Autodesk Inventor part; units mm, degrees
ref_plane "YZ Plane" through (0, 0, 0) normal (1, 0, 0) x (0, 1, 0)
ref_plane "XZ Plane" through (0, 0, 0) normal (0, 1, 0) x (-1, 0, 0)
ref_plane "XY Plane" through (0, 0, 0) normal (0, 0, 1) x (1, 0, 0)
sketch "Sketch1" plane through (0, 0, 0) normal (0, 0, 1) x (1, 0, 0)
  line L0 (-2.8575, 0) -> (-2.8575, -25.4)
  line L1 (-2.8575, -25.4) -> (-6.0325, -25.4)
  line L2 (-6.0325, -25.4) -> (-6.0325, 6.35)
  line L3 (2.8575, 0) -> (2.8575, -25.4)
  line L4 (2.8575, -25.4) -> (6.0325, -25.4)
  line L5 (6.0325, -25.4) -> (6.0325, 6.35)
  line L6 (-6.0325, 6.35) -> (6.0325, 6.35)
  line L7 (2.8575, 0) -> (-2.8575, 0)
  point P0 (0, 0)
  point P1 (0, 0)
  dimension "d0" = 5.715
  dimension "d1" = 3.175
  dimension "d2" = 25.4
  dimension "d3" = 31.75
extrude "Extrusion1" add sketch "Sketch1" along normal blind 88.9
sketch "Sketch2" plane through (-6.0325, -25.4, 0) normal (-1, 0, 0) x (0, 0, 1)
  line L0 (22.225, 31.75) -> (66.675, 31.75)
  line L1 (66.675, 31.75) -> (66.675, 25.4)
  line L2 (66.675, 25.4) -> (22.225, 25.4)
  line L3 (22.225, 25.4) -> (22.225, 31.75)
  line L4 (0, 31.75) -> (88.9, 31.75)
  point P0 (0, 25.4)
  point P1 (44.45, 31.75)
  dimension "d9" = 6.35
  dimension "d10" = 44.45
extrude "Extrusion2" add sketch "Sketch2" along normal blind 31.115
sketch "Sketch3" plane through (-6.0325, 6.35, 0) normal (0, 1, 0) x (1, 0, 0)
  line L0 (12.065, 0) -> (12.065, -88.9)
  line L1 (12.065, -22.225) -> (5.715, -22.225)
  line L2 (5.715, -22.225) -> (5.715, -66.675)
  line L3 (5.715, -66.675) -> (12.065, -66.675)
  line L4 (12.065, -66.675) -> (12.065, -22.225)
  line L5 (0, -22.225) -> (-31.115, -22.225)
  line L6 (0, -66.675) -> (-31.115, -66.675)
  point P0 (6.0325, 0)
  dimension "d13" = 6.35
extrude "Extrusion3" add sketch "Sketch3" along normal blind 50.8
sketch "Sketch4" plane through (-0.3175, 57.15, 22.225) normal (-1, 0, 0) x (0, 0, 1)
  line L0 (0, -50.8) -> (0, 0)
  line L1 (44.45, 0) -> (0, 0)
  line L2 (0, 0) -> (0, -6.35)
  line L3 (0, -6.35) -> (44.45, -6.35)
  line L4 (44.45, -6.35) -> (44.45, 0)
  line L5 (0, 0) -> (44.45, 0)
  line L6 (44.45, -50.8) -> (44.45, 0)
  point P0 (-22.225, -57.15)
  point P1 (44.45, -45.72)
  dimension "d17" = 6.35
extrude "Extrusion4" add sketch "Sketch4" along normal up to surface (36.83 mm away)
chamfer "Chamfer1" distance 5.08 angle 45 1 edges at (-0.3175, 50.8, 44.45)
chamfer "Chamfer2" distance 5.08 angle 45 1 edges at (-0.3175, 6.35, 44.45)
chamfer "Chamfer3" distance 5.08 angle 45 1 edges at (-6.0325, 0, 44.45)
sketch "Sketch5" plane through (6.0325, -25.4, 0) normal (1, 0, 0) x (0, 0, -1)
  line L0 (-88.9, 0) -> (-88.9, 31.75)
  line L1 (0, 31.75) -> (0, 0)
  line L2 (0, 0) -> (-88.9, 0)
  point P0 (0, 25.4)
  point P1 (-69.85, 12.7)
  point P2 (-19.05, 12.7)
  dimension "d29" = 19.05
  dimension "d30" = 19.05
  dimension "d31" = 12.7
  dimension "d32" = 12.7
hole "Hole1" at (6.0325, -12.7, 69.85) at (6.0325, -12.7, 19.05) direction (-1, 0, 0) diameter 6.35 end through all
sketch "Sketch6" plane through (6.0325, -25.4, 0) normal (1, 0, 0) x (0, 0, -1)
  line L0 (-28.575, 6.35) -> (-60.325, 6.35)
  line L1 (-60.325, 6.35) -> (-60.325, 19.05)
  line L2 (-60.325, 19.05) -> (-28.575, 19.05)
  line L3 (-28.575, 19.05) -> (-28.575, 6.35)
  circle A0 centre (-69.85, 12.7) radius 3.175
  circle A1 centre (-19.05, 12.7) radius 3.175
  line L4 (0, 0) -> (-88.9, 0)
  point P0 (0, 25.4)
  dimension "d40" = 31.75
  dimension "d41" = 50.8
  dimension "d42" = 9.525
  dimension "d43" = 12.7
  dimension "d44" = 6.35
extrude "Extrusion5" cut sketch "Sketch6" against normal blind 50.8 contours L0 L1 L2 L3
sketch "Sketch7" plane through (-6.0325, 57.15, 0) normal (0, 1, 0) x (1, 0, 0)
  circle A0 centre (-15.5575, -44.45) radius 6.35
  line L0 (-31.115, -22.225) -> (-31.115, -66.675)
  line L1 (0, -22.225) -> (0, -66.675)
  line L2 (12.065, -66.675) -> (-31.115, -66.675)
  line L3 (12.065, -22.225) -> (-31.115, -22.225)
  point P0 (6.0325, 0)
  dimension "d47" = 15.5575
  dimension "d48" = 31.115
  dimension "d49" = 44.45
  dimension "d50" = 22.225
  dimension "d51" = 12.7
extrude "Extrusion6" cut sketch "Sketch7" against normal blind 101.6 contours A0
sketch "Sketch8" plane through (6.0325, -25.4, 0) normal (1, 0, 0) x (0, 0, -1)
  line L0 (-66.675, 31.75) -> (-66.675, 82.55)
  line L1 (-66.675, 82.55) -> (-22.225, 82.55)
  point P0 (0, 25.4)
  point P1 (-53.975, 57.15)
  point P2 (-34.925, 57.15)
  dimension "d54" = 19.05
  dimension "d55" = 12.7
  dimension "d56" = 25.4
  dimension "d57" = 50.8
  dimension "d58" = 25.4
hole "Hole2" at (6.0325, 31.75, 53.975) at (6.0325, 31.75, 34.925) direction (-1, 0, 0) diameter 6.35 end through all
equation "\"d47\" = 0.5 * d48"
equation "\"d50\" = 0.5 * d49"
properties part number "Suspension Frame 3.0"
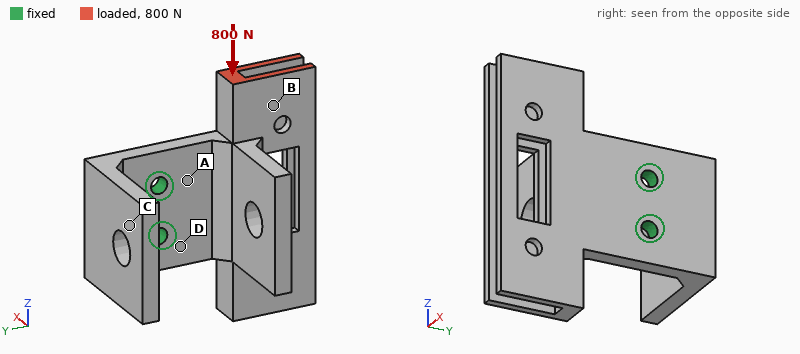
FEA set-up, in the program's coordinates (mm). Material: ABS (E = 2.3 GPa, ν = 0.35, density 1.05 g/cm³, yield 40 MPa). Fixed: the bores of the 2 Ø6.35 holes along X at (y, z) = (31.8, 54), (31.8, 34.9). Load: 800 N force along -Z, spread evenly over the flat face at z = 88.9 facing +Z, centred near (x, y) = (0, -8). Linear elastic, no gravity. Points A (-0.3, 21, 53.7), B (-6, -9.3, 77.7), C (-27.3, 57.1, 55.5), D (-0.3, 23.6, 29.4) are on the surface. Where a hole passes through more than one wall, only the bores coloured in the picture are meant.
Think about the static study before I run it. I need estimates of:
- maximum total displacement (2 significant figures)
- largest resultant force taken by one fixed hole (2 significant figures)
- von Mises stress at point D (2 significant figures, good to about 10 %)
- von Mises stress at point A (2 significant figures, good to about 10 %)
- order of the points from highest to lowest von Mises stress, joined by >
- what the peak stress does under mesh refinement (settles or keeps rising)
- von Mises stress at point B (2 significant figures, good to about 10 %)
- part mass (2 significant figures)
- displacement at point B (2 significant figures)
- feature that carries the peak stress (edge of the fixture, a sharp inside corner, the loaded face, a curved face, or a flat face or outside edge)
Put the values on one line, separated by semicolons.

1.1 mm; 1.4 kN; 8.2 MPa; 11 MPa; A > D > B > C; keeps rising; 4.7 MPa; 54 g; 0.69 mm; edge of the fixture
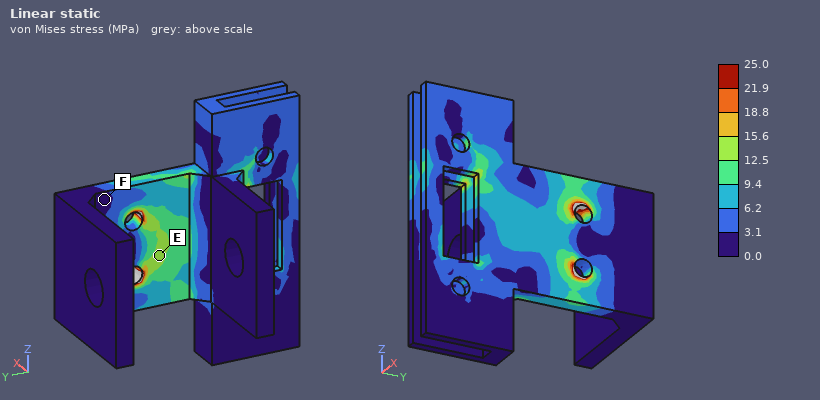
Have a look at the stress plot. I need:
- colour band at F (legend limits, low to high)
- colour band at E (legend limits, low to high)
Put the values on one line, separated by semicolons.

0.0 to 3.1 MPa; 12.5 to 15.6 MPa
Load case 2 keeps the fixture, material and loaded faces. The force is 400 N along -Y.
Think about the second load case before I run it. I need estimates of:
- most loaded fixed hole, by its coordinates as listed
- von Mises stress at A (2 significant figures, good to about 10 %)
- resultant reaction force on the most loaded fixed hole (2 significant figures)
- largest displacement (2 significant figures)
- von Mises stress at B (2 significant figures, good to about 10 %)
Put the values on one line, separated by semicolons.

(31.8, 54); 11 MPa; 980 N; 1.4 mm; 4.4 MPa
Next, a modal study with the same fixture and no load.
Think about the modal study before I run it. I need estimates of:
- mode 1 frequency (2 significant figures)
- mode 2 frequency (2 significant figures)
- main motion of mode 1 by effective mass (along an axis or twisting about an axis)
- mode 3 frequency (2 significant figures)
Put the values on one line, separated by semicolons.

310 Hz; 480 Hz; along X; 600 Hz
